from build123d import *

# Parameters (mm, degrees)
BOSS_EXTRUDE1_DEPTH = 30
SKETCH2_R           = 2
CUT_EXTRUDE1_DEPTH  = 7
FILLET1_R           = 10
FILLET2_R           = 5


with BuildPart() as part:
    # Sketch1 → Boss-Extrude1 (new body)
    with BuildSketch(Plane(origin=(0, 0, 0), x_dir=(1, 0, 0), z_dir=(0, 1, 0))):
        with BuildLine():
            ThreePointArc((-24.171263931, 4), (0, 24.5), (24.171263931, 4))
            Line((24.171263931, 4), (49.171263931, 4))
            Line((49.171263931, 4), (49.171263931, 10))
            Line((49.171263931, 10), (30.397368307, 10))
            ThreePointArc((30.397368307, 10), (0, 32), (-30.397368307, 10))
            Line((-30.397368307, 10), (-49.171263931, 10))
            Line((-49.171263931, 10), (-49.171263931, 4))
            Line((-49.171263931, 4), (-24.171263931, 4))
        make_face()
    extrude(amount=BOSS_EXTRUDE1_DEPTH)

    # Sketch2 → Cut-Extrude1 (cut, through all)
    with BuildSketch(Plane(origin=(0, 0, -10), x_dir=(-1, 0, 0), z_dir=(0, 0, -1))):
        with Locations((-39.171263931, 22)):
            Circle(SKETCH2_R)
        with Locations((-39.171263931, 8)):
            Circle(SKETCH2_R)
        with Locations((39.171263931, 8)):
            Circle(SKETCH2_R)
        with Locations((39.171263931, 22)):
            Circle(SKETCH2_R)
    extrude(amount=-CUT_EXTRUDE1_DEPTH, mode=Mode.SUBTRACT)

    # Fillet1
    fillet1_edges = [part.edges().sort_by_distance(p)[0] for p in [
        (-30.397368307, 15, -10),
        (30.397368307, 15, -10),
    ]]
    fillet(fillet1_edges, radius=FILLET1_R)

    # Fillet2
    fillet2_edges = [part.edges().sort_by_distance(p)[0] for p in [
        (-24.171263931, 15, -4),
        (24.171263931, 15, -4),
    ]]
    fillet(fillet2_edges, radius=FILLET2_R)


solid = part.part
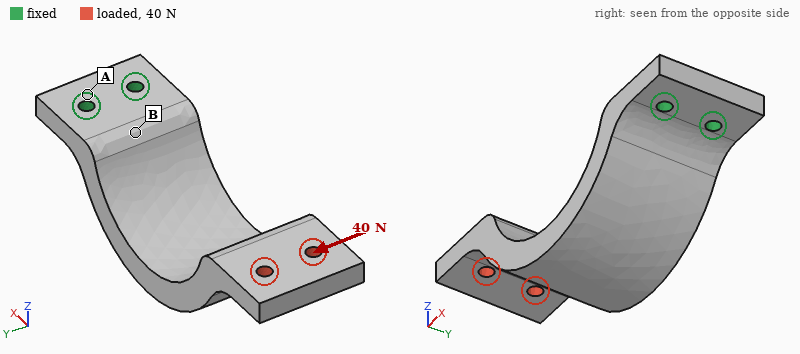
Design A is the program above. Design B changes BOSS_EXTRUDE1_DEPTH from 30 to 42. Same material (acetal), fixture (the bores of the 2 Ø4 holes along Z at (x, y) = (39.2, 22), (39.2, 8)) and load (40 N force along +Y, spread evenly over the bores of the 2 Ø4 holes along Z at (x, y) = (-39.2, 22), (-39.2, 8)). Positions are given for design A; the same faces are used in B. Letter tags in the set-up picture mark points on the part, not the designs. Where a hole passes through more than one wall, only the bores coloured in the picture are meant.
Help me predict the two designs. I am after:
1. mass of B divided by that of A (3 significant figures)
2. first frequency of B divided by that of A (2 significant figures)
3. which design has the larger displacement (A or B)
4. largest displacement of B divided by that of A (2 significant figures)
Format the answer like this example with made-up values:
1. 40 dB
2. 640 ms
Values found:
1. 1.40
2. 0.95
3. A
4. 0.69
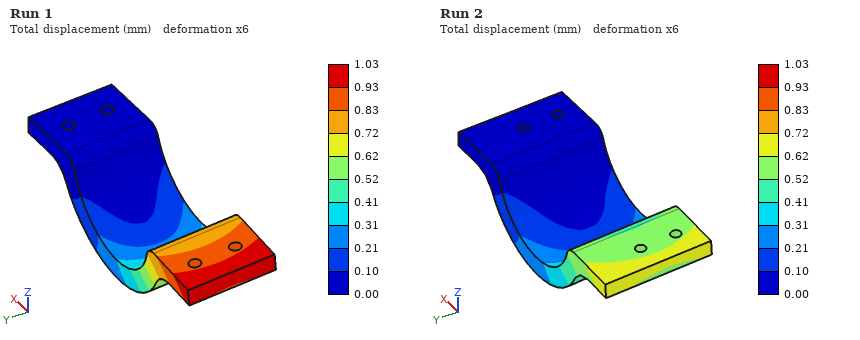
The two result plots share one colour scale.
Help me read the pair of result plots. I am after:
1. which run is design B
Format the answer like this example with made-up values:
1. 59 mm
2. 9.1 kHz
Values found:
1. Run 2
